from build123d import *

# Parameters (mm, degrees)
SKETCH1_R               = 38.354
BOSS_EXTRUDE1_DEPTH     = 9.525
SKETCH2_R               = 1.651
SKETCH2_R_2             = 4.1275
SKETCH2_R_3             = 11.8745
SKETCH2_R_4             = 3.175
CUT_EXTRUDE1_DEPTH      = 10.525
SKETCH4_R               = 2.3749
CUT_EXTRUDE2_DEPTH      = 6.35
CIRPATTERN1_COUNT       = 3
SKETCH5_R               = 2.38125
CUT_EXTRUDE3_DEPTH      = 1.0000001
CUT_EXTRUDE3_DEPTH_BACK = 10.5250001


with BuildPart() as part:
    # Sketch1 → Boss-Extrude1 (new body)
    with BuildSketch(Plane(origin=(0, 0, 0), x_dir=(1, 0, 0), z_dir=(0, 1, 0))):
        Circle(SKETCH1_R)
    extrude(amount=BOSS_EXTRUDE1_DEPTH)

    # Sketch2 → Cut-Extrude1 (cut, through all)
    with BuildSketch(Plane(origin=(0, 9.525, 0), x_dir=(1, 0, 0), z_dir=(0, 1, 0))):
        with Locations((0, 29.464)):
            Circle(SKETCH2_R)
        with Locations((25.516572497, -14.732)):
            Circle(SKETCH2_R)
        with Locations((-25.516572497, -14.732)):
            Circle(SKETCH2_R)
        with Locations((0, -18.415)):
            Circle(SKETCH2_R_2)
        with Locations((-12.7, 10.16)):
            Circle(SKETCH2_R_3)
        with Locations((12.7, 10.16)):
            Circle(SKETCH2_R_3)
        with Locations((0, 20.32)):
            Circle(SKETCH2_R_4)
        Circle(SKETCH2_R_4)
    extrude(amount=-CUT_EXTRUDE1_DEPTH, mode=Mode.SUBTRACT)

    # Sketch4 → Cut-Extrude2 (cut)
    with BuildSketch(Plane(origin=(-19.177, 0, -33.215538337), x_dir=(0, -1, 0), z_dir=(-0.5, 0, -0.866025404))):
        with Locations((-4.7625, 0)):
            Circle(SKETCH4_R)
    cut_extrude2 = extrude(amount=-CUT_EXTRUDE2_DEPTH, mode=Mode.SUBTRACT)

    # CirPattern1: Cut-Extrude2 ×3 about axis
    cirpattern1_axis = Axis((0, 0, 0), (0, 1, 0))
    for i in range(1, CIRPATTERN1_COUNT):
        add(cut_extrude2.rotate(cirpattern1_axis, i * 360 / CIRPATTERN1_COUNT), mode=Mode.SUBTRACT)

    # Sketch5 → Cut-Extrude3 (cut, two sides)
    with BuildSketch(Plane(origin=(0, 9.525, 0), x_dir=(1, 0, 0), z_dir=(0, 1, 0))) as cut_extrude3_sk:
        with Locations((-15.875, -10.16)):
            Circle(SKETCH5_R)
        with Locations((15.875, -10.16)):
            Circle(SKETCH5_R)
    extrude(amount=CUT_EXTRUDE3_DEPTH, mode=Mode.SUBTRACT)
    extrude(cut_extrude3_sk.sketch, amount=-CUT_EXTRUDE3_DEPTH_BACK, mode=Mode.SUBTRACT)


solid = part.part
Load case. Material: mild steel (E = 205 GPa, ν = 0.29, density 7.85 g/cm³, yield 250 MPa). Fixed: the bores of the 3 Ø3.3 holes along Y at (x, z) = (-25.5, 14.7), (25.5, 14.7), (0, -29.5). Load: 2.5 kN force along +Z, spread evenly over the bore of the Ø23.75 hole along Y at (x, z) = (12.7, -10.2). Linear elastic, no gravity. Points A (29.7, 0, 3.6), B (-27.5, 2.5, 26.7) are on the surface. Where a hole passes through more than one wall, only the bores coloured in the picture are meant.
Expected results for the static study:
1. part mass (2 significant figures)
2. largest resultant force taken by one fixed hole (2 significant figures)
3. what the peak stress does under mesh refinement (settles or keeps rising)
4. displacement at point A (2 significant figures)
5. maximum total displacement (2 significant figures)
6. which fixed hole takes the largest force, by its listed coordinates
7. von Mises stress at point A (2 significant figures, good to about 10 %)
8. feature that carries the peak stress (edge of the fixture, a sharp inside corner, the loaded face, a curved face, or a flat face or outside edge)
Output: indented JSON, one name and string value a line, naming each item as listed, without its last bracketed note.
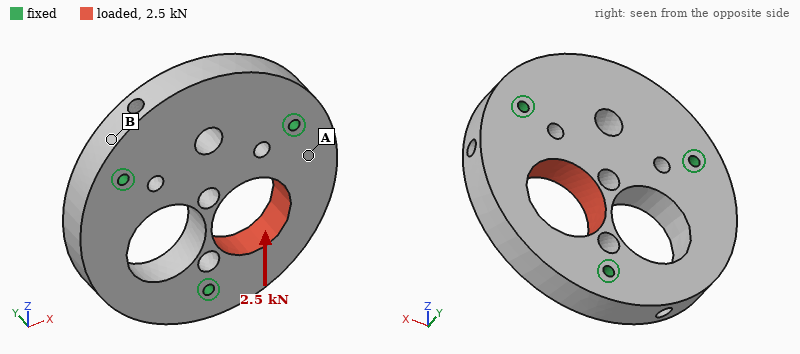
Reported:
{
  "part mass": "260 g",
  "largest resultant force taken by one fixed hole": "1.5 kN",
  "what the peak stress does under mesh refinement": "keeps rising",
  "displacement at point A": "0.57 µm",
  "maximum total displacement": "1.7 µm",
  "which fixed hole takes the largest force, by its listed coordinates": "(25.5, 14.7)",
  "von Mises stress at point A": "7.1 MPa",
  "feature that carries the peak stress": "edge of the fixture"
}
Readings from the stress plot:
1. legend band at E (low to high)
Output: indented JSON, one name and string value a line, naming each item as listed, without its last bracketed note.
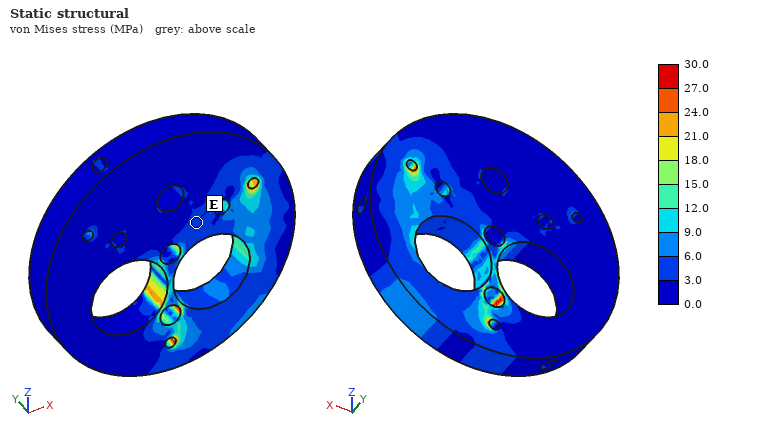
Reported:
{
  "legend band at E": "3.0 to 6.0 MPa"
}
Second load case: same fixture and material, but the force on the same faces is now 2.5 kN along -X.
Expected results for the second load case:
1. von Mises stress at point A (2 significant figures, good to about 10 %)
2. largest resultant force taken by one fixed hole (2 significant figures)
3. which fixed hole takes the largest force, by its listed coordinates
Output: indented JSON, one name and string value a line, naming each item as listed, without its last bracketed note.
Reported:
{
  "von Mises stress at point A": "4.3 MPa",
  "largest resultant force taken by one fixed hole": "1.3 kN",
  "which fixed hole takes the largest force, by its listed coordinates": "(0, -29.5)"
}
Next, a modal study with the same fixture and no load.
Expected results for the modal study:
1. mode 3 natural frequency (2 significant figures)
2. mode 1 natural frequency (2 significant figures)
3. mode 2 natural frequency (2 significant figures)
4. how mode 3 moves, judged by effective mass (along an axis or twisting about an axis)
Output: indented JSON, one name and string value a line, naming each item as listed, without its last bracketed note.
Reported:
{
  "mode 3 natural frequency": "10 kHz",
  "mode 1 natural frequency": "8600 Hz",
  "mode 2 natural frequency": "8800 Hz",
  "how mode 3 moves, judged by effective mass": "along Y"
}
